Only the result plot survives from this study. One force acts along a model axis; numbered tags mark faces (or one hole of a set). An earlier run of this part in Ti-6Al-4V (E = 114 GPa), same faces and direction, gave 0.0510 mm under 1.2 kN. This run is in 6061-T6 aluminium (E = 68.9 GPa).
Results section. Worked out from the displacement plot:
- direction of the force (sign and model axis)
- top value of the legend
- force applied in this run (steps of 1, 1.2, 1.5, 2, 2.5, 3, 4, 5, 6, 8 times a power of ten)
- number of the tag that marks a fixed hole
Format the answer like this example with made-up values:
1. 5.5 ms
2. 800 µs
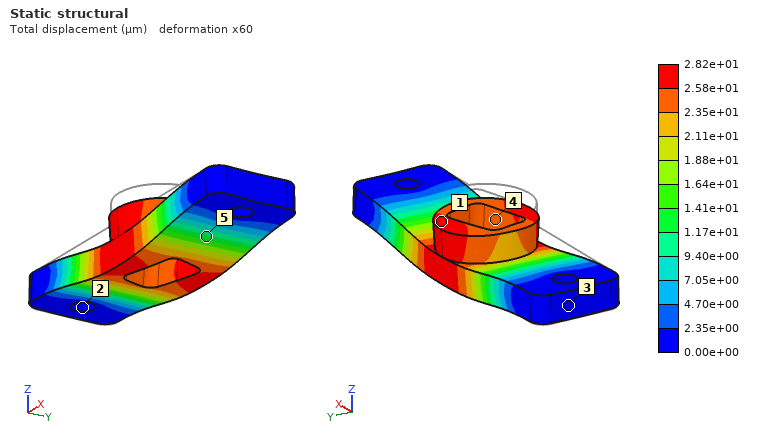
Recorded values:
1. -Z
2. 2.82e+01 µm
3. 400 N
4. 2
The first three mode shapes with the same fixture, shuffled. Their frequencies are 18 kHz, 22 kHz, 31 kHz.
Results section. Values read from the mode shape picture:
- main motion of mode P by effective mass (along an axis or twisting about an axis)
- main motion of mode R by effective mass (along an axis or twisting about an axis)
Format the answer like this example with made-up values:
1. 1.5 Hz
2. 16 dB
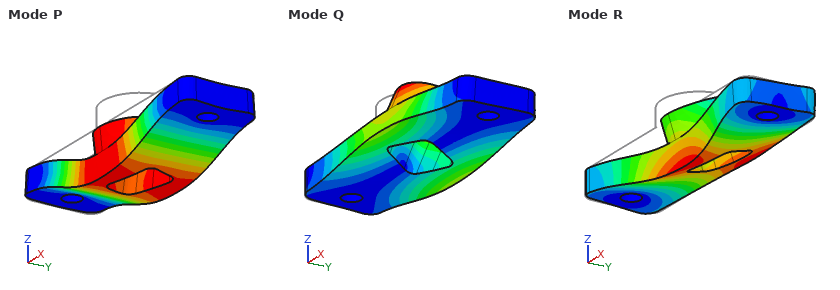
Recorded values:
1. along Z
2. along Y
